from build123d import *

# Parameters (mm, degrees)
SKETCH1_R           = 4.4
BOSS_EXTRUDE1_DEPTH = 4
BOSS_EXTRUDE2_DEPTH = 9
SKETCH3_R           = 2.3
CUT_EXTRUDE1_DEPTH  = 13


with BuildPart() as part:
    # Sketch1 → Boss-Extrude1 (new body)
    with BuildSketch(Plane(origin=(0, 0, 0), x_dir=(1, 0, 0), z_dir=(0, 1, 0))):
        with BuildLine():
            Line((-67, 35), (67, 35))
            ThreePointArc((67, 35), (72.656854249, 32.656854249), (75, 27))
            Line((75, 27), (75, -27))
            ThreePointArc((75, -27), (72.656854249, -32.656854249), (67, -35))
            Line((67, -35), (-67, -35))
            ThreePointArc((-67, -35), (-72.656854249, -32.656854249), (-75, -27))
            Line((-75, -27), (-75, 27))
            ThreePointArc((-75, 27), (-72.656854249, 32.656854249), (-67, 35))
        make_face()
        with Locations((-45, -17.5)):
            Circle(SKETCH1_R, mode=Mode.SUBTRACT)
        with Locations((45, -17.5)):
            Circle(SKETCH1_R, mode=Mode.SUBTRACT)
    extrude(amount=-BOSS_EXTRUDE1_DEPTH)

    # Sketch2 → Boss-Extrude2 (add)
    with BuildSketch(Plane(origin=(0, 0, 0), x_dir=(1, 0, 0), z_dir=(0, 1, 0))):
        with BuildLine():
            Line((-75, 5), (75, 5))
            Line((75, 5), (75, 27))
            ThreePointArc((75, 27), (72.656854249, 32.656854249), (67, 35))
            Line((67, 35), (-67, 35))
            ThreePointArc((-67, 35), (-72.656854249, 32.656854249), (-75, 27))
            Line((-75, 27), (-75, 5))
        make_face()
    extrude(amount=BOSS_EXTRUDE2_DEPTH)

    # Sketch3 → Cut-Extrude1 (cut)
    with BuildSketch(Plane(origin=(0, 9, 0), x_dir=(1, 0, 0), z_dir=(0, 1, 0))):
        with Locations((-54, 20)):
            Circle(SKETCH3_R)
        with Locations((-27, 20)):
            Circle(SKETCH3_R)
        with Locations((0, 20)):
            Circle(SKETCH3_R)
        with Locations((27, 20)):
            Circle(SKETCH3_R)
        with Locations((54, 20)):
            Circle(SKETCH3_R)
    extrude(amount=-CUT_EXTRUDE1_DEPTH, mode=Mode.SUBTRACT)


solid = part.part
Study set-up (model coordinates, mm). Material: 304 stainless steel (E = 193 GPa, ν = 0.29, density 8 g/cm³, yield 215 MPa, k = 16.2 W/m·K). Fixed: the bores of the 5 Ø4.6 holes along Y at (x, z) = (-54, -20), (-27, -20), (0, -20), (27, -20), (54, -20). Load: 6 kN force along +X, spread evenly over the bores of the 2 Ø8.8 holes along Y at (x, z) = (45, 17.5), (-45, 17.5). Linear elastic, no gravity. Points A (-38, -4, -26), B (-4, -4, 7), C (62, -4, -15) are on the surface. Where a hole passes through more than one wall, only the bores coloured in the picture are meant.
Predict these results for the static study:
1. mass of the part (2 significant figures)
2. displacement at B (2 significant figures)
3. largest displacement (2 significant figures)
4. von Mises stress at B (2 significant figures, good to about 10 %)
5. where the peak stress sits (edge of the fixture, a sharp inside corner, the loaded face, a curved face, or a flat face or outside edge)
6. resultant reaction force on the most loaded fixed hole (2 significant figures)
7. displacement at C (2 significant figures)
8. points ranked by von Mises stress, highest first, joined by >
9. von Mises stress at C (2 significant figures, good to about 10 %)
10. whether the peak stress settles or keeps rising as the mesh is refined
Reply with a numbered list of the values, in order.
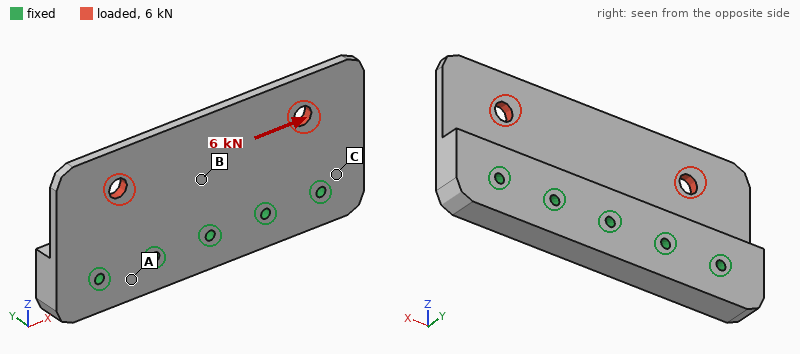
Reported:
1. 640 g
2. 2.7 µm
3. 8.3 µm
4. 17 MPa
5. a sharp inside corner
6. 2.4 kN
7. 1.3 µm
8. B > C > A
9. 8.1 MPa
10. keeps rising
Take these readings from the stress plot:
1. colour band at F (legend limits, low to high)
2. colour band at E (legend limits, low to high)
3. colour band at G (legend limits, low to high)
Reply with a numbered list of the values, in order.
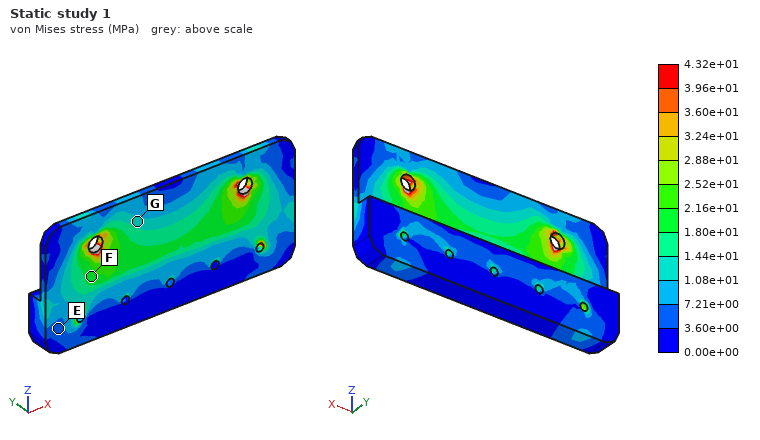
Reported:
1. 1.80e+01 to 2.16e+01 MPa
2. 3.60e+00 to 7.21e+00 MPa
3. 1.08e+01 to 1.44e+01 MPa
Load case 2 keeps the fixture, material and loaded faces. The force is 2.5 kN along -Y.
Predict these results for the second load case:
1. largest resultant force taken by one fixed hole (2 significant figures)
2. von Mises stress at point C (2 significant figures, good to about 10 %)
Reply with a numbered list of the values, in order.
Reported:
1. 700 N
2. 20 MPa
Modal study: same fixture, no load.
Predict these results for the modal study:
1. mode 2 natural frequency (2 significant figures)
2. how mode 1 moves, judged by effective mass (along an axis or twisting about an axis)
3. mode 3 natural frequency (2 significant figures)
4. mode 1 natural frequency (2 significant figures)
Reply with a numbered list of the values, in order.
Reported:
1. 2200 Hz
2. along Y
3. 3000 Hz
4. 1800 Hz
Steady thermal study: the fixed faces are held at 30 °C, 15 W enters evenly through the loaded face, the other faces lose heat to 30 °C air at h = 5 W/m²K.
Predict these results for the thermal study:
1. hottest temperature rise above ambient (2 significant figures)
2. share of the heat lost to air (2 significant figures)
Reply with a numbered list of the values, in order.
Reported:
1. 69 K
2. 15 %
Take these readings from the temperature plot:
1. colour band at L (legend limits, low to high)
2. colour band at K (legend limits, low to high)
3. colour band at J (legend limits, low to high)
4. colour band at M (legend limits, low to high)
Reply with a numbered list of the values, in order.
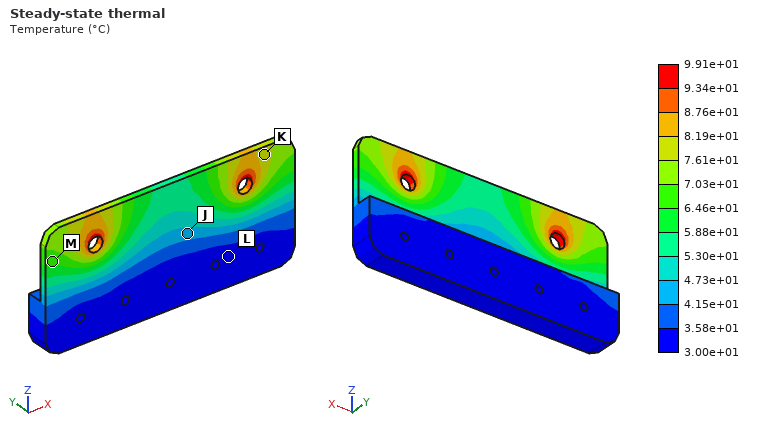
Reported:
1. 3.00e+01 to 3.58e+01 °C
2. 7.61e+01 to 8.19e+01 °C
3. 4.15e+01 to 4.73e+01 °C
4. 6.46e+01 to 7.03e+01 °C
